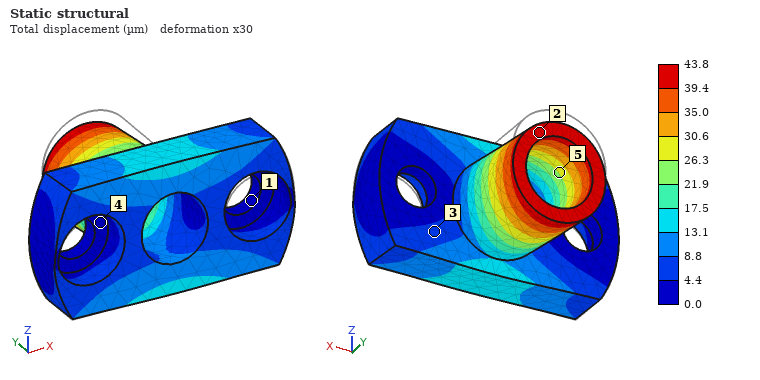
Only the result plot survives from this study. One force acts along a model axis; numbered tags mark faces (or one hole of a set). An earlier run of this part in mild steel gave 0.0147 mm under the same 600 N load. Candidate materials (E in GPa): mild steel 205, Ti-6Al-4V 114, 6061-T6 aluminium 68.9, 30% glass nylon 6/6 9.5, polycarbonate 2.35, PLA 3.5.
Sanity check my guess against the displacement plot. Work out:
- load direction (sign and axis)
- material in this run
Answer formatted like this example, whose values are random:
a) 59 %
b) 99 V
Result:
a) -Z
b) 6061-T6 aluminium
